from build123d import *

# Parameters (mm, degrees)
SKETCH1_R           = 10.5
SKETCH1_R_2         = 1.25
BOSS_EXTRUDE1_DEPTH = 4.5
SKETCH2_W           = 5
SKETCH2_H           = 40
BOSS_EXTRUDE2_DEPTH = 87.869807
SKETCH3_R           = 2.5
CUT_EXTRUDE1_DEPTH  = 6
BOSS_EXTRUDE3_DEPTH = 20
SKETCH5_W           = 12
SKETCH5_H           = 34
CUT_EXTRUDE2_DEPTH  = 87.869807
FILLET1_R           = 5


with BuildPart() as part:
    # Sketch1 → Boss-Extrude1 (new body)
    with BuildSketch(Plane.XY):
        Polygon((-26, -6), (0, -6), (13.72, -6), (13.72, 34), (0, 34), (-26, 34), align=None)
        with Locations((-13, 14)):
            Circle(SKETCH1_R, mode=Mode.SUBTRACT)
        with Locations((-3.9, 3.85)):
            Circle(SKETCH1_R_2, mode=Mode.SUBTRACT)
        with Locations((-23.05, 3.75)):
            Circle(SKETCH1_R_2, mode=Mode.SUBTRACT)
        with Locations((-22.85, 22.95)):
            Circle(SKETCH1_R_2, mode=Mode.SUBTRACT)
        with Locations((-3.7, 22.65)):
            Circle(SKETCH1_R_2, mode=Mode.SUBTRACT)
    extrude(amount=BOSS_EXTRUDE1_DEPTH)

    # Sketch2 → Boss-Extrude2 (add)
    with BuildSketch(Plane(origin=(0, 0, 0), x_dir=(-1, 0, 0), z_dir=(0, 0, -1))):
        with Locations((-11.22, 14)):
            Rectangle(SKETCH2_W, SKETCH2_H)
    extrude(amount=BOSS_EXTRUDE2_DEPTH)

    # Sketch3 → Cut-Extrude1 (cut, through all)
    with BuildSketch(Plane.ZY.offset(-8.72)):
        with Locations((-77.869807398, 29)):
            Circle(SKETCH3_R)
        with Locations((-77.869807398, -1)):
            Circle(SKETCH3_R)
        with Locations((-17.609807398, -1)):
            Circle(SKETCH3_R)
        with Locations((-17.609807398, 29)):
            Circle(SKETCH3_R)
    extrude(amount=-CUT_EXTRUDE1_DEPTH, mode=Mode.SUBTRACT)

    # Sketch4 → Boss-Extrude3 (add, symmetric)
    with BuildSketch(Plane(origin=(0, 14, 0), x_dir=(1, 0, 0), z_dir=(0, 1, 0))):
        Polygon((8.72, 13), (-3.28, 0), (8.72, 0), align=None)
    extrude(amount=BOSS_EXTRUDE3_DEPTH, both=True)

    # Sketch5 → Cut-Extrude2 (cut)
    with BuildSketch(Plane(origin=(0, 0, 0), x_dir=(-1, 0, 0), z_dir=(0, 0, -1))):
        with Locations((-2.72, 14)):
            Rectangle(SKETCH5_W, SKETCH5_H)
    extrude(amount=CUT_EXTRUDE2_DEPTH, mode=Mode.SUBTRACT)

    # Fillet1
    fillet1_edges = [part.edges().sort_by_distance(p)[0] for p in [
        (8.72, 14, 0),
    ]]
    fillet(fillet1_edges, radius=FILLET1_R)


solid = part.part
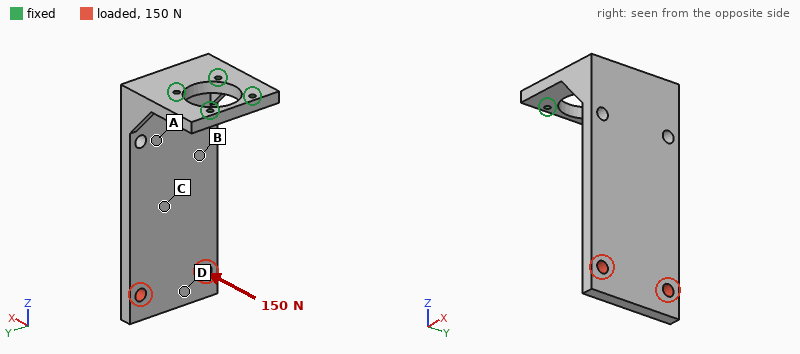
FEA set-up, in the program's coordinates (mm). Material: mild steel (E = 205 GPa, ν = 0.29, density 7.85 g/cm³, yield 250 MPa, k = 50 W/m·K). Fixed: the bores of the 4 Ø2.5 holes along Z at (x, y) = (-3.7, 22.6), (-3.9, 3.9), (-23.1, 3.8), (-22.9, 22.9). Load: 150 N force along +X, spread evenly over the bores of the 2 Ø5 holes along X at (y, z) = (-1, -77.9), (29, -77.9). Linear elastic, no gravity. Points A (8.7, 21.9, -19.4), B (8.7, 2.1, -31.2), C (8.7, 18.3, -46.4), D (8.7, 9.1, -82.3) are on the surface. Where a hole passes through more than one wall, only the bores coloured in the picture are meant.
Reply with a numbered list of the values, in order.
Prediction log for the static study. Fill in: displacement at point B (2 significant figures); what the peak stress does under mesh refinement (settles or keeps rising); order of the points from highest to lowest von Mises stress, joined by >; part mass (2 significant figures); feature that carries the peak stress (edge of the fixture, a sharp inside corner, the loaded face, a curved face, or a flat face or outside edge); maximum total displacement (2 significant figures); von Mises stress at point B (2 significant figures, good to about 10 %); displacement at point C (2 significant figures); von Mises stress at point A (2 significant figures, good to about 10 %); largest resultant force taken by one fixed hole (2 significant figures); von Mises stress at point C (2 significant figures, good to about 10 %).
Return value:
1. 0.11 mm
2. keeps rising
3. A > B > C > D
4. 180 g
5. edge of the fixture
6. 0.48 mm
7. 42 MPa
8. 0.20 mm
9. 60 MPa
10. 140 N
11. 28 MPa
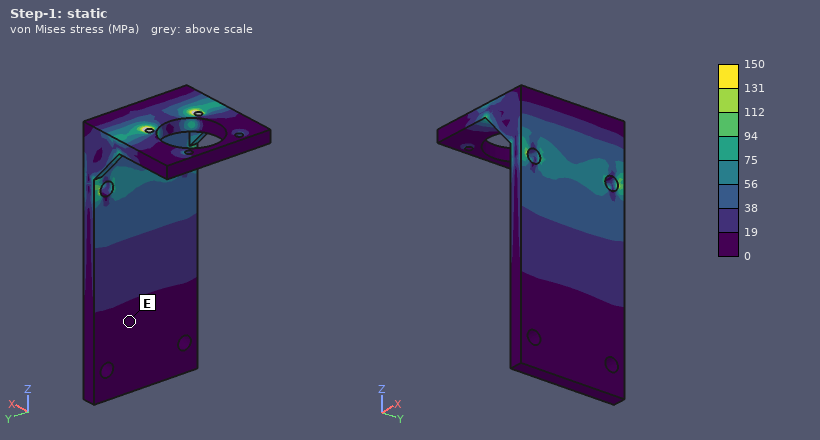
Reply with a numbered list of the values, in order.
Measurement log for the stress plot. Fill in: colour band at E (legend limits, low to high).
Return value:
1. 0 to 19 MPa
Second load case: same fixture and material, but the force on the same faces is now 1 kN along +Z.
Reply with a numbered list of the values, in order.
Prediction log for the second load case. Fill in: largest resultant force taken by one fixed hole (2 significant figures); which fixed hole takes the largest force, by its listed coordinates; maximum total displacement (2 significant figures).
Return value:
1. 650 N
2. (-3.7, 22.6)
3. 0.17 mm
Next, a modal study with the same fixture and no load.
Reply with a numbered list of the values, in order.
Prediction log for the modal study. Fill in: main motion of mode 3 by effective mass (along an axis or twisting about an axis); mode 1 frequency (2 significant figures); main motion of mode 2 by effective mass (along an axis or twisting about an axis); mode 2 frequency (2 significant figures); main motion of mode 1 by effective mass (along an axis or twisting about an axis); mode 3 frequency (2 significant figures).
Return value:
1. along Z
2. 430 Hz
3. along Y
4. 1100 Hz
5. along X
6. 2400 Hz
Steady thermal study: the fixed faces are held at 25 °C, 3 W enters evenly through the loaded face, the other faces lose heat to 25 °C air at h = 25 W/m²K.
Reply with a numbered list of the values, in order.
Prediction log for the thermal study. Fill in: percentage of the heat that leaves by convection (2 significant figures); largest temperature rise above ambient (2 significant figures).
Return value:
1. 61 %
2. 17 K
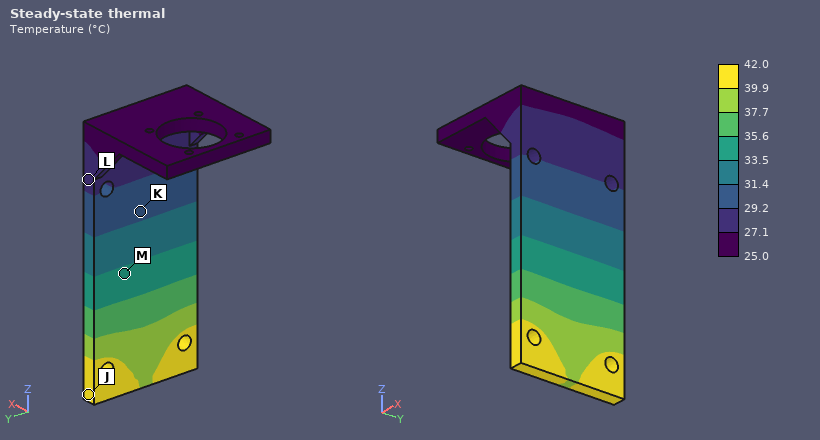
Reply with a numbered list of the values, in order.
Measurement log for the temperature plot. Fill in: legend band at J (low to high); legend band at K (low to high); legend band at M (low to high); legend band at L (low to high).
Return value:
1. 39.9 to 42.0 °C
2. 29.2 to 31.4 °C
3. 33.5 to 35.6 °C
4. 27.1 to 29.2 °C
